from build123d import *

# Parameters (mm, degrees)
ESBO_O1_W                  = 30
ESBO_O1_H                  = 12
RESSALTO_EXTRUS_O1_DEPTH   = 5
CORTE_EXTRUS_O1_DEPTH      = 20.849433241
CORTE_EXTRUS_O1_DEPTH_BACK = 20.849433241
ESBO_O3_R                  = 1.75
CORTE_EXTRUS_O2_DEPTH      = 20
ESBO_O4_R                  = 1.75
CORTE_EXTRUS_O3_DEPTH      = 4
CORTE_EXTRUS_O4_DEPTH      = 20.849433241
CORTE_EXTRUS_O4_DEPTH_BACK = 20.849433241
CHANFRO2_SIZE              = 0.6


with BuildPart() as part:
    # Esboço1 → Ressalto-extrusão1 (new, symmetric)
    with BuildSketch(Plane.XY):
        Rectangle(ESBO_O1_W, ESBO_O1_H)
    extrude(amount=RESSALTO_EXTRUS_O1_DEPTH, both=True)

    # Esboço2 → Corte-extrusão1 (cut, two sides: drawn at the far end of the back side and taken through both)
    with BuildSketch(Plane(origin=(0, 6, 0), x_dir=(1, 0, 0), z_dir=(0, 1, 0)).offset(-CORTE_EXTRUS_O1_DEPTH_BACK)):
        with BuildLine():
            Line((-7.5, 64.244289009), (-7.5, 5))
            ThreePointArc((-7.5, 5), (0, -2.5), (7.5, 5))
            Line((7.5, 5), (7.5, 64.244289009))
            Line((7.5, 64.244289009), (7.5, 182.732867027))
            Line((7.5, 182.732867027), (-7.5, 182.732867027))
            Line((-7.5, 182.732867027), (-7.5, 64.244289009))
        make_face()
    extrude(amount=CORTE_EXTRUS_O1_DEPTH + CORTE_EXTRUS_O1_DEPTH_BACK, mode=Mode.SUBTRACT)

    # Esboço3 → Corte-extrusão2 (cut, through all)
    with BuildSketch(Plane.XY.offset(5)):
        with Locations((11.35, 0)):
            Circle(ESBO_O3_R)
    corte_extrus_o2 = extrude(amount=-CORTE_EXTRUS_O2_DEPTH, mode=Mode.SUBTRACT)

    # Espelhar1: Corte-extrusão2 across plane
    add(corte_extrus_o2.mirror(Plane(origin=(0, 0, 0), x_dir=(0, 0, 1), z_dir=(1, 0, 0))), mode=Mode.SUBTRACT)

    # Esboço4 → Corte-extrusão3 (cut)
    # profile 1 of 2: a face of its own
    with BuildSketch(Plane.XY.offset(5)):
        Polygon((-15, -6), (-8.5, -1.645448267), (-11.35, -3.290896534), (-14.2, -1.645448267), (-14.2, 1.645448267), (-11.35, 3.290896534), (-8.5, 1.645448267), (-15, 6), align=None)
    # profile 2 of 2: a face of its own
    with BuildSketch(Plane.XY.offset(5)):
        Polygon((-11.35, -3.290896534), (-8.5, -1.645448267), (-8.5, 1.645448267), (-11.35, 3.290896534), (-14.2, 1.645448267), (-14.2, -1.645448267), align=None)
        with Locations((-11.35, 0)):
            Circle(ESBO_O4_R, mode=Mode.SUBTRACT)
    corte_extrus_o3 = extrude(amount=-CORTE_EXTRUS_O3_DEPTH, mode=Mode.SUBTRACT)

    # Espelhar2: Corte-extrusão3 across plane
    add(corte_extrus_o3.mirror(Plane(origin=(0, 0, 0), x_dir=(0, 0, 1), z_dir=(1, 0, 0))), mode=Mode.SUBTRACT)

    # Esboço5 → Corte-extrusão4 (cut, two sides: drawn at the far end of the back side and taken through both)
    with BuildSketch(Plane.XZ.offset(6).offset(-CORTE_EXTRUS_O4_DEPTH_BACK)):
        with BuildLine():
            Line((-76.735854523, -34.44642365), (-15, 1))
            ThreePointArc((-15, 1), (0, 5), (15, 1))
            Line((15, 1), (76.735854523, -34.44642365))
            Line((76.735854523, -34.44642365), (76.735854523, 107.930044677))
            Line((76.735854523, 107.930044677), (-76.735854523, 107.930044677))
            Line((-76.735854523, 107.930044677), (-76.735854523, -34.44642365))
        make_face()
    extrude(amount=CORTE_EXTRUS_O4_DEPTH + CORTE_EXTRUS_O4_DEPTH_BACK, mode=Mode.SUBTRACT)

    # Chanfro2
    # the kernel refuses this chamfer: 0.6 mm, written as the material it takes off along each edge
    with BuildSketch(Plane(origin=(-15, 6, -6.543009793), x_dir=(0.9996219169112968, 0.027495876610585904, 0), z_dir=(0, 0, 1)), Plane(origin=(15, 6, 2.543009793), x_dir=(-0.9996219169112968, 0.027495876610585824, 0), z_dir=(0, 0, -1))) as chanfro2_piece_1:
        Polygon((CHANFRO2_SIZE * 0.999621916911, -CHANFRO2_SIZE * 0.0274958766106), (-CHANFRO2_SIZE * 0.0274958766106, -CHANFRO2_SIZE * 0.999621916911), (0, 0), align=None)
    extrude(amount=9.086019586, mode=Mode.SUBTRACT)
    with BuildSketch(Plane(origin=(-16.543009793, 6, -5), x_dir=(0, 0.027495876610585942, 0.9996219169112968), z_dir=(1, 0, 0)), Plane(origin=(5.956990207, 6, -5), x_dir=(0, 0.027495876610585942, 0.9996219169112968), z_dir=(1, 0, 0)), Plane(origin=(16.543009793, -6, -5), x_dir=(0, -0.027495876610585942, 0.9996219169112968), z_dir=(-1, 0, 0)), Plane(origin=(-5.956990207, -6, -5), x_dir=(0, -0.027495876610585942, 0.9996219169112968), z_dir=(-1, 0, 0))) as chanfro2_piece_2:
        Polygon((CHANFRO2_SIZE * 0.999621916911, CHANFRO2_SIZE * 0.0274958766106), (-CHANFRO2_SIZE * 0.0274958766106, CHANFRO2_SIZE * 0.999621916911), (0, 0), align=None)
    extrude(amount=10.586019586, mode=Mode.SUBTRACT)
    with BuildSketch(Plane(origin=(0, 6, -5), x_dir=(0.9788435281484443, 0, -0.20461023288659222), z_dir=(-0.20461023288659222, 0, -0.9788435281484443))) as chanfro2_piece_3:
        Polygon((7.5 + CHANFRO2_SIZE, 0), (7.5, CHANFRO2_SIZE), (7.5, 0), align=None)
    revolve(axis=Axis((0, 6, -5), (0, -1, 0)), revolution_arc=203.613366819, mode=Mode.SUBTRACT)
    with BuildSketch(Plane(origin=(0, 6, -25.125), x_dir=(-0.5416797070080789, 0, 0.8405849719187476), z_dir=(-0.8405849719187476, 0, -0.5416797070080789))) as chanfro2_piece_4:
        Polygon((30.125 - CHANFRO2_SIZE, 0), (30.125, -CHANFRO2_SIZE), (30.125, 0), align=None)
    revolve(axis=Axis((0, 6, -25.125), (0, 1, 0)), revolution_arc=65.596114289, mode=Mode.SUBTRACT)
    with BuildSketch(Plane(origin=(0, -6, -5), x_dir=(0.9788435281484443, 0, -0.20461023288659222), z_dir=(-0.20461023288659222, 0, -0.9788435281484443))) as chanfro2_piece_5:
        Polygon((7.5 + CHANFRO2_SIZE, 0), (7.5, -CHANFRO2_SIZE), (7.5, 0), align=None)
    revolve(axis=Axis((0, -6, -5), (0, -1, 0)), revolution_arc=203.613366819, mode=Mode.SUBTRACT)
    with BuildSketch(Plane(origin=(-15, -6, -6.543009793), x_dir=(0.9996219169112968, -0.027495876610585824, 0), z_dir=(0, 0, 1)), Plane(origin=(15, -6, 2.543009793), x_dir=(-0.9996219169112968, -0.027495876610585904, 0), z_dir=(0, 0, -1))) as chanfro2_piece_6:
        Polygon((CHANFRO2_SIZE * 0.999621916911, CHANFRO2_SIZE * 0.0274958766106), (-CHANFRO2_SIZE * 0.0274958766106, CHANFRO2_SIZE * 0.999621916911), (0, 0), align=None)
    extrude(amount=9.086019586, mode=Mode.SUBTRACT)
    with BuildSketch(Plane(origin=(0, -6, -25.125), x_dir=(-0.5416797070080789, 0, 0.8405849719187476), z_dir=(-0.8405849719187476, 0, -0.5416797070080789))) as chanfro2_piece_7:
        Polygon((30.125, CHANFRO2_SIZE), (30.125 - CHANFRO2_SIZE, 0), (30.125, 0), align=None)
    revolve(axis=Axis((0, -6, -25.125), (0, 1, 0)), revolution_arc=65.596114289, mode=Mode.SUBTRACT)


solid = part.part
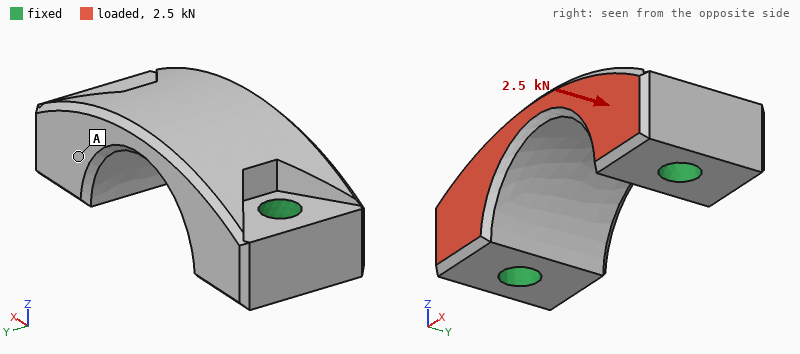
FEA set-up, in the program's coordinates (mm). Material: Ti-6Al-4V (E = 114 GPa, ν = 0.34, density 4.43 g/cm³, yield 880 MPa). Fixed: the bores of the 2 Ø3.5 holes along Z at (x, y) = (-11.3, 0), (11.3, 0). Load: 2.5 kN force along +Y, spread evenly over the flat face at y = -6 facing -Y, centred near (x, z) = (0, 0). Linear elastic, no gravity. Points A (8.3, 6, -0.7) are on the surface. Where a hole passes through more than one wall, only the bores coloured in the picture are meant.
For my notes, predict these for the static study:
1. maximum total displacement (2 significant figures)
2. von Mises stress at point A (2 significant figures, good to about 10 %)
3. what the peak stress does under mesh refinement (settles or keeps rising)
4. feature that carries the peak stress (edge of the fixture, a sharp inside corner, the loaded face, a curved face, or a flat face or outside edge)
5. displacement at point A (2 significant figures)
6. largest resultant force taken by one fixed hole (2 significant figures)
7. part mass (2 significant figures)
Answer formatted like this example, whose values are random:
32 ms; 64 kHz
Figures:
6.4 µm; 14 MPa; keeps rising; edge of the fixture; 2.1 µm; 1.3 kN; 8.0 g
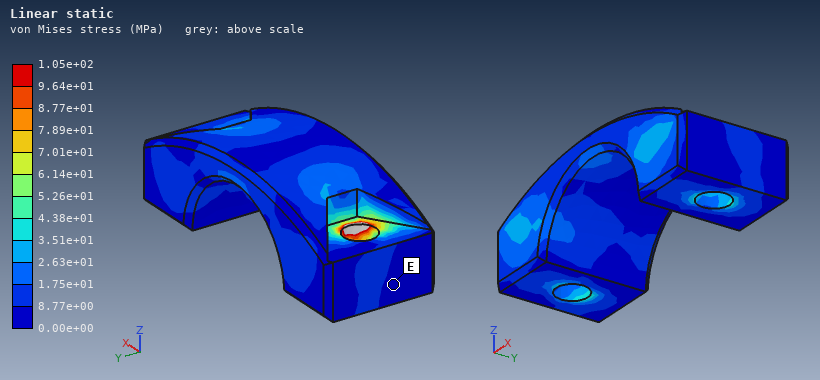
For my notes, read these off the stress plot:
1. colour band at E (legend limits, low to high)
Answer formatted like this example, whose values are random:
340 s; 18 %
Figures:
0.00e+00 to 8.77e+00 MPa
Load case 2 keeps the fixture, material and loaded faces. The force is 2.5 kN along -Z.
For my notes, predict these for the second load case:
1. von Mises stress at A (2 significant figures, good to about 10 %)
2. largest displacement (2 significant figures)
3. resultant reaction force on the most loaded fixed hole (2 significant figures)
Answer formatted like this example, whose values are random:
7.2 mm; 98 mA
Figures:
22 MPa; 14 µm; 1.3 kN
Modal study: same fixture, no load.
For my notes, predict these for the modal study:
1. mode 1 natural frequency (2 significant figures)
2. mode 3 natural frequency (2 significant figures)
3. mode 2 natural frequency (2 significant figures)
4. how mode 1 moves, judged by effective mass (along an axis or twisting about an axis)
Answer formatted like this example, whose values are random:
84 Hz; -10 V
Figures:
39 kHz; 60 kHz; 59 kHz; along Y
